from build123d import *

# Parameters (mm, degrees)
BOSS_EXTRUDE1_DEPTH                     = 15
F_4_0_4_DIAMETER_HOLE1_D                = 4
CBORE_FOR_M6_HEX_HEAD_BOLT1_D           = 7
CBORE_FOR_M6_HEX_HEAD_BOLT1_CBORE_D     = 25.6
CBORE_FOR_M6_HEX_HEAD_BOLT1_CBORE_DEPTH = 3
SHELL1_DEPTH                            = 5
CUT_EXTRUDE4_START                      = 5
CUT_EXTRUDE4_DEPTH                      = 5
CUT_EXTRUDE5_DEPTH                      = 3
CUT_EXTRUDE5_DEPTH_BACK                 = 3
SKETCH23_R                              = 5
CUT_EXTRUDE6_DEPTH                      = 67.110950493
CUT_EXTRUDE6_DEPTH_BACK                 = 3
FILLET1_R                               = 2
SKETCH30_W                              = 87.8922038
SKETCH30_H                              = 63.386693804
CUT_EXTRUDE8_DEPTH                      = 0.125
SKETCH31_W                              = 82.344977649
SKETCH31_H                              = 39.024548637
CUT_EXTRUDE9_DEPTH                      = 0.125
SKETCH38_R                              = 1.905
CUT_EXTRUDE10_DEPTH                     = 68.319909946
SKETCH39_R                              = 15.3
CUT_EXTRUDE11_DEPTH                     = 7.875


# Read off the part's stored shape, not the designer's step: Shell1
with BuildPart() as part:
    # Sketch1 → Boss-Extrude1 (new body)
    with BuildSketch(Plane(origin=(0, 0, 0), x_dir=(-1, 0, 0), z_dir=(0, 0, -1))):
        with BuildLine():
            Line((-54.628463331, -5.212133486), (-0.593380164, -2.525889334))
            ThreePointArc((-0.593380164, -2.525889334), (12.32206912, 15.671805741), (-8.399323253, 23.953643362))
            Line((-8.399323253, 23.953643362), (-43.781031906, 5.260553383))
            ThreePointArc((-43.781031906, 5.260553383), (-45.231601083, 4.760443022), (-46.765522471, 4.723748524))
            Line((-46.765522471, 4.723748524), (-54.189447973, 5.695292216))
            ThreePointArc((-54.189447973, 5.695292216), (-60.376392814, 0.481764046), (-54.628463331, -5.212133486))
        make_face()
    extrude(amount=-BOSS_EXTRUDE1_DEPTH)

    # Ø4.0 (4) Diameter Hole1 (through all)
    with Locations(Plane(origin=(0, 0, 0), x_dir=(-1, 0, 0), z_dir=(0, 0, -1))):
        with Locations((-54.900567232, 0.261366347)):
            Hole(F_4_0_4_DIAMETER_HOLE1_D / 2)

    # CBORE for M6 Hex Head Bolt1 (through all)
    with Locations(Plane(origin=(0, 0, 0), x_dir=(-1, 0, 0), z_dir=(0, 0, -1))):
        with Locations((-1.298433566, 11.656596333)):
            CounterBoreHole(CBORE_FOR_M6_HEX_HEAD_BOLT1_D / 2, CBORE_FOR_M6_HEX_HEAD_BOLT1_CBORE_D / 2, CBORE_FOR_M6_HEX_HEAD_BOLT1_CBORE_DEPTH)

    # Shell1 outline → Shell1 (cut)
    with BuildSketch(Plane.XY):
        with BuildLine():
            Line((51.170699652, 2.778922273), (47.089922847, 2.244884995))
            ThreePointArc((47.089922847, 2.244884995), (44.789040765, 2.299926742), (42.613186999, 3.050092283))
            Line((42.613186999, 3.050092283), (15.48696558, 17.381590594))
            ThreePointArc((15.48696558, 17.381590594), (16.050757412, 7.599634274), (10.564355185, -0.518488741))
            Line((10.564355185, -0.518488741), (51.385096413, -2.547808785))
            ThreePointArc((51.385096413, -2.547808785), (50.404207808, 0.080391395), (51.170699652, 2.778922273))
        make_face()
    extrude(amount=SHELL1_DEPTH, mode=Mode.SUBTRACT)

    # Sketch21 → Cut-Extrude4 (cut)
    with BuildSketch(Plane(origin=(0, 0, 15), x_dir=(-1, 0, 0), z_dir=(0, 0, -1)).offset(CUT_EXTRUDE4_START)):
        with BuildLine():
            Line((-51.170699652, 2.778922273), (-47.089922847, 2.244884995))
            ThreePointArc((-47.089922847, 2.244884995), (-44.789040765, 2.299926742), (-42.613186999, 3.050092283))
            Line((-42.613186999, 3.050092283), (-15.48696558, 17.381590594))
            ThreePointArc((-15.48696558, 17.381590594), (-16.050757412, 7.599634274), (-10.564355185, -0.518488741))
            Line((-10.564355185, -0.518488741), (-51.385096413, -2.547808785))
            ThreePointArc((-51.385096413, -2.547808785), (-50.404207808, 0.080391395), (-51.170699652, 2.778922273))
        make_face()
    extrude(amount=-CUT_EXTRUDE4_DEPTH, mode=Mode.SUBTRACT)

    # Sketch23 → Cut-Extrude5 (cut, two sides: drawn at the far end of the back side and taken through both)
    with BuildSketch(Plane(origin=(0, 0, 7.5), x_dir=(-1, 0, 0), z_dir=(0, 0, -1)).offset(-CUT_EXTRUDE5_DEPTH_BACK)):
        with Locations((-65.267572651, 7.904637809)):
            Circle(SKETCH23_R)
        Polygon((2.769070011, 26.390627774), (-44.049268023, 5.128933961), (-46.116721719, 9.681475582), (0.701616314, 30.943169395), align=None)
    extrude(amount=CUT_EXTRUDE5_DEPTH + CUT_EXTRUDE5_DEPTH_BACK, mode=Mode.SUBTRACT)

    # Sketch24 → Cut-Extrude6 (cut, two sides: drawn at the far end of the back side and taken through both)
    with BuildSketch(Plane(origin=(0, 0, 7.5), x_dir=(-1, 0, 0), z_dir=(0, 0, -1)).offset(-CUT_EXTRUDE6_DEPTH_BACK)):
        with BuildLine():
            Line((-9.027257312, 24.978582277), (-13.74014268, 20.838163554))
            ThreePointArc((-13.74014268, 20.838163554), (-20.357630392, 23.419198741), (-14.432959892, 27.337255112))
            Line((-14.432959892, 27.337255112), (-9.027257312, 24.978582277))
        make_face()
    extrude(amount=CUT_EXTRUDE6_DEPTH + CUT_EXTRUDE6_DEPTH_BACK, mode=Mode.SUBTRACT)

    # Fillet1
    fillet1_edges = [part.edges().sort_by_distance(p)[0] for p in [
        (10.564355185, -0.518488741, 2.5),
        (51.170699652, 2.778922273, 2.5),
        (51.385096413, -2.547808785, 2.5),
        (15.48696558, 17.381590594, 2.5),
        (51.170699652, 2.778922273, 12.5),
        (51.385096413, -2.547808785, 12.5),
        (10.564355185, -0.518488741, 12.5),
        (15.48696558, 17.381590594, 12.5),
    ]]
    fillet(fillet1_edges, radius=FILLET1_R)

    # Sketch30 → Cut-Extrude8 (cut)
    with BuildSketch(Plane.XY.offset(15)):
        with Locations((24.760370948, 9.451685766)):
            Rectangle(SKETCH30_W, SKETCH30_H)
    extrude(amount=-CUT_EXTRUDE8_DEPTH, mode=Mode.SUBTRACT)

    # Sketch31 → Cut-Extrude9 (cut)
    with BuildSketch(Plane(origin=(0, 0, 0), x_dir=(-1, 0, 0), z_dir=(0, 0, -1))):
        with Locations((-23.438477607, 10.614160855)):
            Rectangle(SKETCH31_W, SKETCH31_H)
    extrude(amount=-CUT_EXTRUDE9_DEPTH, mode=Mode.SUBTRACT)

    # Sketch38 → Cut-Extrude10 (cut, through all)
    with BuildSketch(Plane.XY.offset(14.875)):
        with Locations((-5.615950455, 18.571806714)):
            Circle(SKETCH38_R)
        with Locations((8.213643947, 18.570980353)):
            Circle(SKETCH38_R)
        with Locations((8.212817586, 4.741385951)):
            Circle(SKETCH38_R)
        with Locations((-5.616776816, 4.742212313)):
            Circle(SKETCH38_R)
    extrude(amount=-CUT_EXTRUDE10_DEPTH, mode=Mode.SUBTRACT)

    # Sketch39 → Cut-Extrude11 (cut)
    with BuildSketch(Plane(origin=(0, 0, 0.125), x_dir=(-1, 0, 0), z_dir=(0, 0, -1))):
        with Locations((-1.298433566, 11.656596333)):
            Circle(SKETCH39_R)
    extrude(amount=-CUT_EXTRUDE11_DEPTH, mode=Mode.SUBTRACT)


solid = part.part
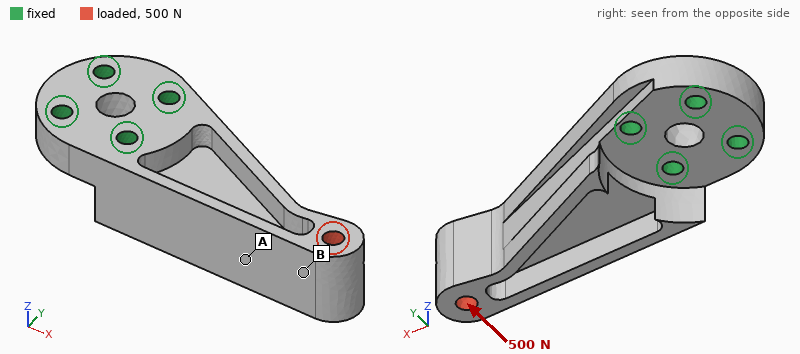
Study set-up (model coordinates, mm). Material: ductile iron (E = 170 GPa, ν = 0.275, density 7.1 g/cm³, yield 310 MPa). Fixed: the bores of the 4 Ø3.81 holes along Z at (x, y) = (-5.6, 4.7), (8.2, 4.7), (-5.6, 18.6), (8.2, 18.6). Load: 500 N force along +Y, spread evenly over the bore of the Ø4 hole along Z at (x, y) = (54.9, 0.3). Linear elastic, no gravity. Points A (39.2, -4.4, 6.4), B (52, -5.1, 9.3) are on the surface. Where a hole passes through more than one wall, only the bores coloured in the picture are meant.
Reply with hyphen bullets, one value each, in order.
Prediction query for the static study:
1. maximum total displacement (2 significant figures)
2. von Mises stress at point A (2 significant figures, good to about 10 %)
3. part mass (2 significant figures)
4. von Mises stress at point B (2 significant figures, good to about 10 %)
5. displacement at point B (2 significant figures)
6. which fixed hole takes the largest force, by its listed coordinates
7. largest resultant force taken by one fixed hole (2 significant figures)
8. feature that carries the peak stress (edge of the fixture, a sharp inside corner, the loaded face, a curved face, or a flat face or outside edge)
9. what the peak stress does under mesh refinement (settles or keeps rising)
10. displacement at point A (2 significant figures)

- 43 µm
- 29 MPa
- 70 g
- 7.0 MPa
- 32 µm
- (8.2, 18.6)
- 1.3 kN
- a sharp inside corner
- keeps rising
- 16 µm
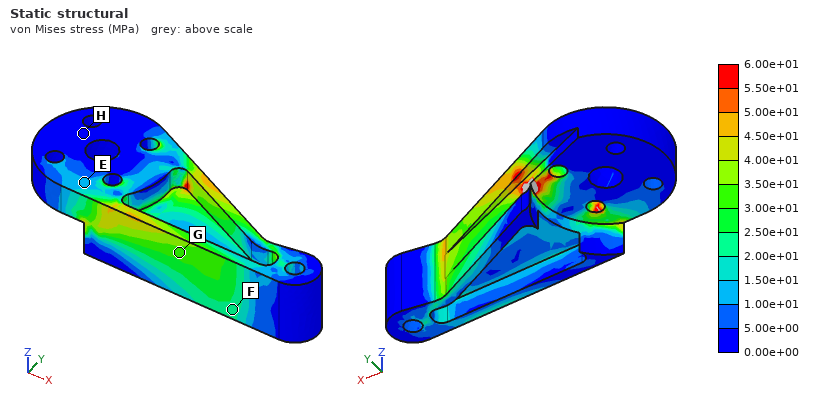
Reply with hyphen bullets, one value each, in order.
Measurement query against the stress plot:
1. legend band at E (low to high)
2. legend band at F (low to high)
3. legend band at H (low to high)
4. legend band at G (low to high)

- 1.00e+01 to 1.50e+01 MPa
- 2.00e+01 to 2.50e+01 MPa
- 0.00e+00 to 5.00e+00 MPa
- 3.00e+01 to 3.50e+01 MPa
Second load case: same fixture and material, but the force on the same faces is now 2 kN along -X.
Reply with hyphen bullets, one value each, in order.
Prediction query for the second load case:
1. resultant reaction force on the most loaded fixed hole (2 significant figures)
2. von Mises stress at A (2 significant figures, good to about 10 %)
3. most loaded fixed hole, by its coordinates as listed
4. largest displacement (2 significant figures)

- 1.8 kN
- 24 MPa
- (8.2, 4.7)
- 41 µm
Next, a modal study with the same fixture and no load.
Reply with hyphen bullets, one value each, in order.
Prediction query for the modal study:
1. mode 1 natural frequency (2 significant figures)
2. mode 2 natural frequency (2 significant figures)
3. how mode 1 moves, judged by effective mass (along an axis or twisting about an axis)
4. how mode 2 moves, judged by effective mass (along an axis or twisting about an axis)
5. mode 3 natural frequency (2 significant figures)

- 2100 Hz
- 5200 Hz
- along Z
- along Y
- 8800 Hz
